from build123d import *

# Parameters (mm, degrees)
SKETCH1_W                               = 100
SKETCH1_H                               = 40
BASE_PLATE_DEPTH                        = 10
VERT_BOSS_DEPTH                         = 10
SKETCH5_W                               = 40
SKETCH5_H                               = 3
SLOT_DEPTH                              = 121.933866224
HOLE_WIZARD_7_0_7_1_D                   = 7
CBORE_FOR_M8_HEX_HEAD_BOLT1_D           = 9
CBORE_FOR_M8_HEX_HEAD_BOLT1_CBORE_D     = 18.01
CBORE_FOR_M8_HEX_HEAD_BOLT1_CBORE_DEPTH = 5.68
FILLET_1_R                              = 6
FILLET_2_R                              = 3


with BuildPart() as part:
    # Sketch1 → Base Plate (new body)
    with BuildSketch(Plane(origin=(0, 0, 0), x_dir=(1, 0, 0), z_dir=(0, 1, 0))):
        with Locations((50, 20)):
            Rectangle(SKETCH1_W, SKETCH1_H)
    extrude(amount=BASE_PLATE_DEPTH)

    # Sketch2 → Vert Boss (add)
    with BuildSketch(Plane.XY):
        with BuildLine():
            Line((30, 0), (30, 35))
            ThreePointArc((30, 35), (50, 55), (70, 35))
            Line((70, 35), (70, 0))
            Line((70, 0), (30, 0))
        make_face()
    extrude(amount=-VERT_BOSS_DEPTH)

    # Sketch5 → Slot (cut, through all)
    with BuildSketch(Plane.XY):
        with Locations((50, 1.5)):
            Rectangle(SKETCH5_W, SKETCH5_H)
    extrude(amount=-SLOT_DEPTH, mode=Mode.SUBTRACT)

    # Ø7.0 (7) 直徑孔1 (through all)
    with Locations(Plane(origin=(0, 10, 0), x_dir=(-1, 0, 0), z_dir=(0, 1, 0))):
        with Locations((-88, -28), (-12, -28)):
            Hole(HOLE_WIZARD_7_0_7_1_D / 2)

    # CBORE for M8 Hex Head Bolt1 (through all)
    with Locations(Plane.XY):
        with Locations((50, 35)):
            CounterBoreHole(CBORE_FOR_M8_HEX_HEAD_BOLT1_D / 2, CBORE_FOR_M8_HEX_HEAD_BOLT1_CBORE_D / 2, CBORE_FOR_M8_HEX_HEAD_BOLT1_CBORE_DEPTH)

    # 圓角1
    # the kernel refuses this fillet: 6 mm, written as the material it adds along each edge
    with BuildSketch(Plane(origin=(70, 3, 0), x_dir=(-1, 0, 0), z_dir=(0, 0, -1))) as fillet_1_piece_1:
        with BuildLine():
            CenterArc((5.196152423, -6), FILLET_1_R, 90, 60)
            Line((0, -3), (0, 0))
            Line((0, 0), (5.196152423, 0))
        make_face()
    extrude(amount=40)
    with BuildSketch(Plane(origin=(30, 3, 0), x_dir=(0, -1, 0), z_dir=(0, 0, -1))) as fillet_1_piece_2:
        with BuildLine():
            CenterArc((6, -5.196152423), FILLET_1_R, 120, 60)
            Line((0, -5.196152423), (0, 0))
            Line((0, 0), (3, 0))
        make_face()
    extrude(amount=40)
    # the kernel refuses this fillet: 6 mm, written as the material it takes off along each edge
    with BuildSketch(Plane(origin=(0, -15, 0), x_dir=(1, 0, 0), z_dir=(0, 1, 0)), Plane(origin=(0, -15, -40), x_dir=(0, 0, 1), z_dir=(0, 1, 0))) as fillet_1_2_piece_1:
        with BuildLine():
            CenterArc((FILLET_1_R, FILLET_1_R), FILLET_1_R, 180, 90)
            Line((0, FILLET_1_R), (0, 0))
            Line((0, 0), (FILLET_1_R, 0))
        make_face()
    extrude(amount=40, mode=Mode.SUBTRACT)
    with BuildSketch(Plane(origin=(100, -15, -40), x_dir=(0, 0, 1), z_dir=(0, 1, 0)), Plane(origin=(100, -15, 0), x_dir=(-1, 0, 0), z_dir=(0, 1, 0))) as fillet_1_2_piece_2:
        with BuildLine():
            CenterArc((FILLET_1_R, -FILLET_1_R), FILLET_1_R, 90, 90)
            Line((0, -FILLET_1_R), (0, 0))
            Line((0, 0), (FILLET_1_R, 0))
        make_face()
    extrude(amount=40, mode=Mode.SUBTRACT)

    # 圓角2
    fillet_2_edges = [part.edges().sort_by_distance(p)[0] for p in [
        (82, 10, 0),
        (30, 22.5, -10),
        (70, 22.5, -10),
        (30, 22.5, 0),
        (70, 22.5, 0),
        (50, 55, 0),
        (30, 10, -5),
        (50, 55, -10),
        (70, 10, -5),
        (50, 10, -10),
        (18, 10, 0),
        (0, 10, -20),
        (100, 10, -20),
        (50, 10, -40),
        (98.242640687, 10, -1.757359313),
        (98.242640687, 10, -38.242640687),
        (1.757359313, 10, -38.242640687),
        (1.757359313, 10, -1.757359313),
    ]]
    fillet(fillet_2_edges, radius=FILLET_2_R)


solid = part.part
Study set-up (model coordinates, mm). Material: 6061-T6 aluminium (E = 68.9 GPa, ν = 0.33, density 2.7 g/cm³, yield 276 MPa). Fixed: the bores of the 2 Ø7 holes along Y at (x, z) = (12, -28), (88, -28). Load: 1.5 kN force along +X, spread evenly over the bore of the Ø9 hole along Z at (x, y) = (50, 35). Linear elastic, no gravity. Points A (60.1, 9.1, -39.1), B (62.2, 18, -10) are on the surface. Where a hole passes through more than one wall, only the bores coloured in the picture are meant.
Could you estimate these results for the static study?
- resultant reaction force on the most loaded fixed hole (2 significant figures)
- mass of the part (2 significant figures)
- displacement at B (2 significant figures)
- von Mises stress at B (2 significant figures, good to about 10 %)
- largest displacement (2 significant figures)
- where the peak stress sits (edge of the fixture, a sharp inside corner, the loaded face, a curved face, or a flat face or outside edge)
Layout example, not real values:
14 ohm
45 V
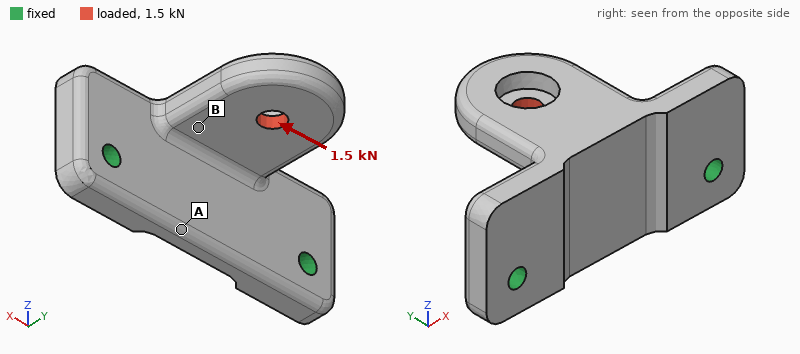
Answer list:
1.1 kN
130 g
19 µm
21 MPa
61 µm
a curved face
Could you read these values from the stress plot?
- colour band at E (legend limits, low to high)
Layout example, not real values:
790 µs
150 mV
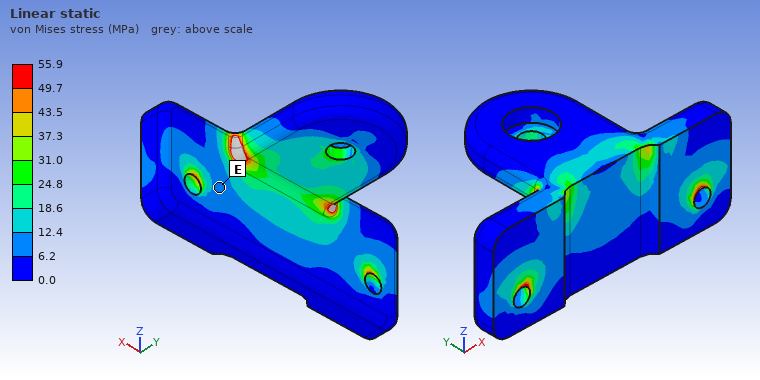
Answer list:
6.2 to 12.4 MPa
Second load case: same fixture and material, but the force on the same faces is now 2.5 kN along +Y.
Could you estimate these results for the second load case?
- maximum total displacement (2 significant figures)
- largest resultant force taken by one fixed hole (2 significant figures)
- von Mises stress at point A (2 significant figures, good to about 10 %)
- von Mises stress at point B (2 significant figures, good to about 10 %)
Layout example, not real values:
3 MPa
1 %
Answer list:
97 µm
1.3 kN
8.2 MPa
21 MPa
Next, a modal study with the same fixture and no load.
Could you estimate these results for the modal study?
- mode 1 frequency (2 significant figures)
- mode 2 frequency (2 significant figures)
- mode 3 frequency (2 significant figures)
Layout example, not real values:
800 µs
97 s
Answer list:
2300 Hz
5000 Hz
5100 Hz
